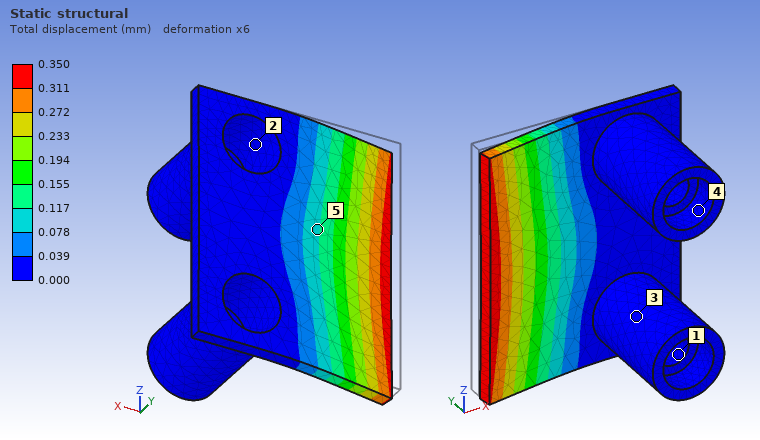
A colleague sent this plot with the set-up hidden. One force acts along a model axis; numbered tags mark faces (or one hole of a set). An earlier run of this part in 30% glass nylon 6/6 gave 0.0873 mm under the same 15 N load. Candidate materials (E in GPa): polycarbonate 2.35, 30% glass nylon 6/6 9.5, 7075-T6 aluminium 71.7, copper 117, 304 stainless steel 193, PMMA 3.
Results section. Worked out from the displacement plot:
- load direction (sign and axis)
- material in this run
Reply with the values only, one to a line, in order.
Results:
-Y
polycarbonate
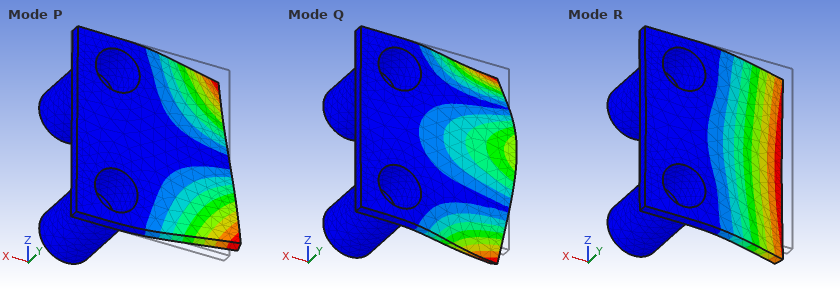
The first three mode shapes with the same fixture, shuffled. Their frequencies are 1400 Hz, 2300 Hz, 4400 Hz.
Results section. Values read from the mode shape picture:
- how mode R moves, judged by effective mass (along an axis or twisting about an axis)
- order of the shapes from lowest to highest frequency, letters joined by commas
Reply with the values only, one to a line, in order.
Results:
along Y
R, P, Q
